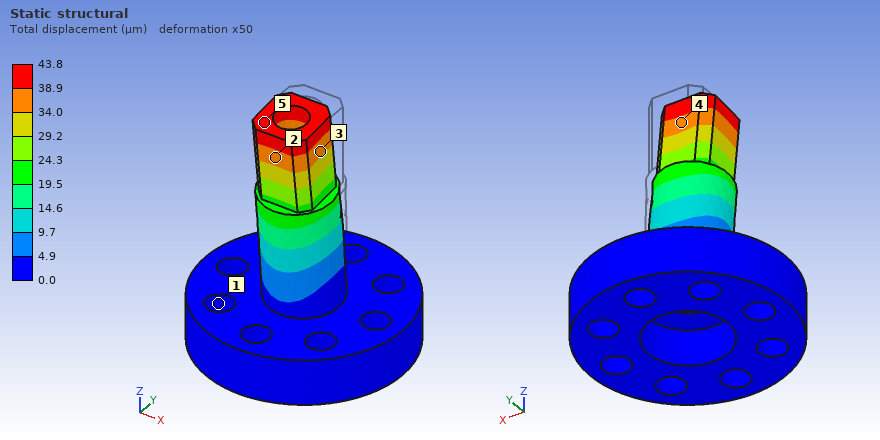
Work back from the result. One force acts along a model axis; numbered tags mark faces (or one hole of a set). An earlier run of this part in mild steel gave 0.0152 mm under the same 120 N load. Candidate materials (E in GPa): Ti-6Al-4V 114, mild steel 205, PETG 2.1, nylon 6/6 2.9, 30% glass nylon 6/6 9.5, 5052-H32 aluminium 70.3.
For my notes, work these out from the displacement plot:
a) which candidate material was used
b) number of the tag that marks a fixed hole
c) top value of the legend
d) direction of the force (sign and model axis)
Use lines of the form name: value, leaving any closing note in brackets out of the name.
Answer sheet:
which candidate material was used: 5052-H32 aluminium
number of the tag that marks a fixed hole: 1
top value of the legend: 43.8 µm
direction of the force: -Y
